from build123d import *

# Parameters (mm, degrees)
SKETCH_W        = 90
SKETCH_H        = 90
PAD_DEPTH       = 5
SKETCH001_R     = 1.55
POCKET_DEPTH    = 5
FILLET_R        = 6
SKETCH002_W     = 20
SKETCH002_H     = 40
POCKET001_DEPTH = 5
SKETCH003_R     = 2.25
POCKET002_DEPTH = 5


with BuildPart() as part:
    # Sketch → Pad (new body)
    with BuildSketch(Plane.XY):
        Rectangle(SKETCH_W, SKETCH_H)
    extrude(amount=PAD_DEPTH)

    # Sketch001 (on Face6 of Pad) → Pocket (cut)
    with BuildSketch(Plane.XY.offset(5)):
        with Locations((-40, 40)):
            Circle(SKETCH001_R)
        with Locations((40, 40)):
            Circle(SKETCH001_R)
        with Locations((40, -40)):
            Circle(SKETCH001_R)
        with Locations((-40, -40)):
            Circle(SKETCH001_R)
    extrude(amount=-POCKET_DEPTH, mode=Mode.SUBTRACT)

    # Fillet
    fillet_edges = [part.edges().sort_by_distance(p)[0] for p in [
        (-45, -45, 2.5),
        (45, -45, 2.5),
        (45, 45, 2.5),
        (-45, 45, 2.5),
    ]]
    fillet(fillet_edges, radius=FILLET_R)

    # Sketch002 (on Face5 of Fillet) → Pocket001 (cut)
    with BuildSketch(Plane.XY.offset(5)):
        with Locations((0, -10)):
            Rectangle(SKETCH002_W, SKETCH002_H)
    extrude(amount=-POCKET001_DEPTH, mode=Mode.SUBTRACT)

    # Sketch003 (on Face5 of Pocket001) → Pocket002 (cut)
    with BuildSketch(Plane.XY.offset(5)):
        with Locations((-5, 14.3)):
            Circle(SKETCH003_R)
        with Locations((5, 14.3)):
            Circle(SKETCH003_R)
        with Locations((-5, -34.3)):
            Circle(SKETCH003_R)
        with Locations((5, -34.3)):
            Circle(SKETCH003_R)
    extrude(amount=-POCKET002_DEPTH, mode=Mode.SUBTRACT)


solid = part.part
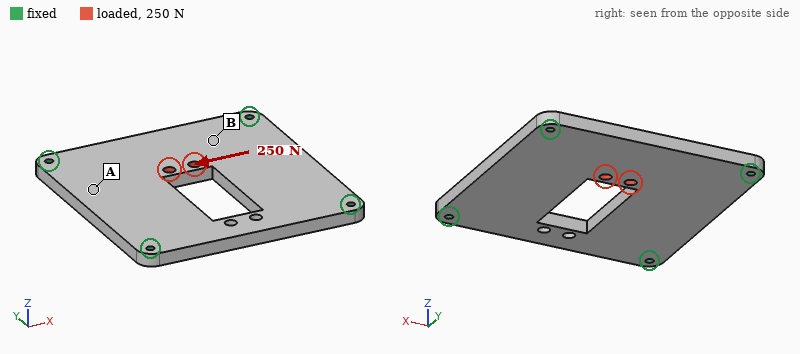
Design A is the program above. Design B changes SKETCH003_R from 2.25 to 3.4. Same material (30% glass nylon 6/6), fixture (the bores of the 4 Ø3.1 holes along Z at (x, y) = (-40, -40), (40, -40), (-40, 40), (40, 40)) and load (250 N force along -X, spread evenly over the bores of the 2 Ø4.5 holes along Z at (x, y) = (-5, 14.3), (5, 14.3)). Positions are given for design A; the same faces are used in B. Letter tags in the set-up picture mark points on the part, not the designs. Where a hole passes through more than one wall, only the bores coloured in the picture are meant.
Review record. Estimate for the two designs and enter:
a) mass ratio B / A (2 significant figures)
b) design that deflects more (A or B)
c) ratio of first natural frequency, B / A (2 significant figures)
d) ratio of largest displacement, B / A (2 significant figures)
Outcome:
0.99
B
0.99
1.3
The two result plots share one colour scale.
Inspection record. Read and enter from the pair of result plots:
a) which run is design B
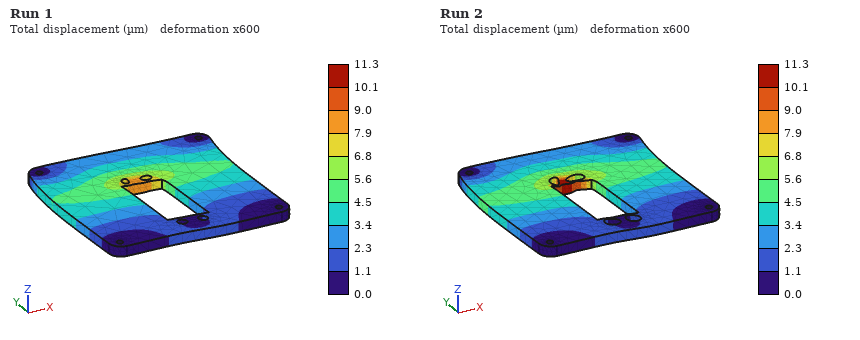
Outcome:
Run 2
